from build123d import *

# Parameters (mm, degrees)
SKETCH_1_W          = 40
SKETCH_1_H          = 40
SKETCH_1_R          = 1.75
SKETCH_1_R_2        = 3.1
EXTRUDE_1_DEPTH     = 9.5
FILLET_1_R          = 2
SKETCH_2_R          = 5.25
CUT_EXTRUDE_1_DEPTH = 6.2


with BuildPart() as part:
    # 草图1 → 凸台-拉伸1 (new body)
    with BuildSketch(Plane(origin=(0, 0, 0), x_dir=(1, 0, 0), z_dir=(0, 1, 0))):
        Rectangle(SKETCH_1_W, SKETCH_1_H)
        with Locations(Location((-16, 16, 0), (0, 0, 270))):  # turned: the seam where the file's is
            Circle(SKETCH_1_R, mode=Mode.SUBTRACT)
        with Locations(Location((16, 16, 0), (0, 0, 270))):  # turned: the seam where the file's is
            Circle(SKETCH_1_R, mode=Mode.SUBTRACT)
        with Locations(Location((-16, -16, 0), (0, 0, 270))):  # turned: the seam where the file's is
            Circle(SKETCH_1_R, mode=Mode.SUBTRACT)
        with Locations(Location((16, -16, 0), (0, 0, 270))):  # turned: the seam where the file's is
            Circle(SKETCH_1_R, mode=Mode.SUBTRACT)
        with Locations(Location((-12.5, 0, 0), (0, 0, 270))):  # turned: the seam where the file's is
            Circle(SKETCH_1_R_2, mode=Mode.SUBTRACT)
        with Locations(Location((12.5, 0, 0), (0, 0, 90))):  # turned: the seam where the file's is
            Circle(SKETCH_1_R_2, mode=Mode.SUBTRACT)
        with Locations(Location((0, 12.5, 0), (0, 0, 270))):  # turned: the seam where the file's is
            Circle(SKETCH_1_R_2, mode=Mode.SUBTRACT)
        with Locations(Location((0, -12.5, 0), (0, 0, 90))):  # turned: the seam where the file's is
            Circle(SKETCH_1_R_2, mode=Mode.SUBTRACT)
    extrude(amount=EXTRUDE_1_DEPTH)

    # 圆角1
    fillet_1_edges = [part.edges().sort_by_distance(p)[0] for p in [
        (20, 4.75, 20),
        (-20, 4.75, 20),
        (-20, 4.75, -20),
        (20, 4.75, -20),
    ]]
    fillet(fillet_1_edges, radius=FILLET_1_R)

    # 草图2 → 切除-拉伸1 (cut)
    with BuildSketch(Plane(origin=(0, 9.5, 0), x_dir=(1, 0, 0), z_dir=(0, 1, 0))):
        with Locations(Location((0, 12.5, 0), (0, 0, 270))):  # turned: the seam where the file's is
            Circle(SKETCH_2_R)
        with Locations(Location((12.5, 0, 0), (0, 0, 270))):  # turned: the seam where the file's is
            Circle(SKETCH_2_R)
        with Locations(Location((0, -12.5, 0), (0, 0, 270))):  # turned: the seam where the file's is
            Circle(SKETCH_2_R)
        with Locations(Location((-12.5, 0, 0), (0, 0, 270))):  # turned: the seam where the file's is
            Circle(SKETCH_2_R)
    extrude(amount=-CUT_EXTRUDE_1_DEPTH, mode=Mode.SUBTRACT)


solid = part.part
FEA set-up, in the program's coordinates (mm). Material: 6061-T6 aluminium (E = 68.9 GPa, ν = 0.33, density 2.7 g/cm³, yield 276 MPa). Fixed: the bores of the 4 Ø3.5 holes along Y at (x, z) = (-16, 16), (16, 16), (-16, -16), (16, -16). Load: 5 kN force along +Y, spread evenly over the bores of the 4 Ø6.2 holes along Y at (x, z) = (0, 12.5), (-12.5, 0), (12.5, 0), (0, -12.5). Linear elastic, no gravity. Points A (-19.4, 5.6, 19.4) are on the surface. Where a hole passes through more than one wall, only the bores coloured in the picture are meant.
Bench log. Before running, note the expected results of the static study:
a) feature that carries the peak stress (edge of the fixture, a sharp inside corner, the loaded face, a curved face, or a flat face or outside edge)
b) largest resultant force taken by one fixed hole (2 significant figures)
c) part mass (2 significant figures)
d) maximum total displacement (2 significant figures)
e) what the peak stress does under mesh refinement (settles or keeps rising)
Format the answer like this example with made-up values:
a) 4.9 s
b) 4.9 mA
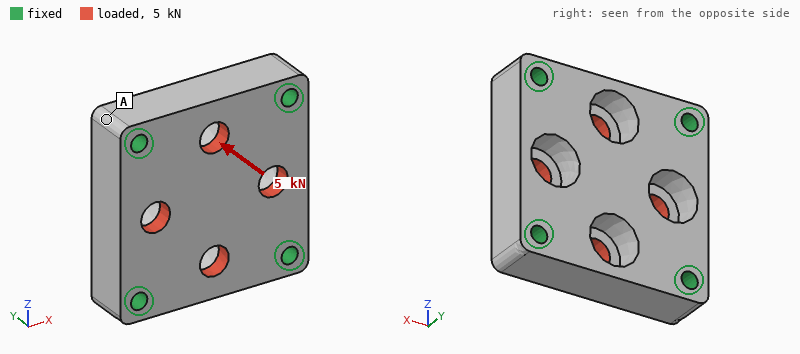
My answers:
a) edge of the fixture
b) 1.3 kN
c) 33 g
d) 16 µm
e) keeps rising
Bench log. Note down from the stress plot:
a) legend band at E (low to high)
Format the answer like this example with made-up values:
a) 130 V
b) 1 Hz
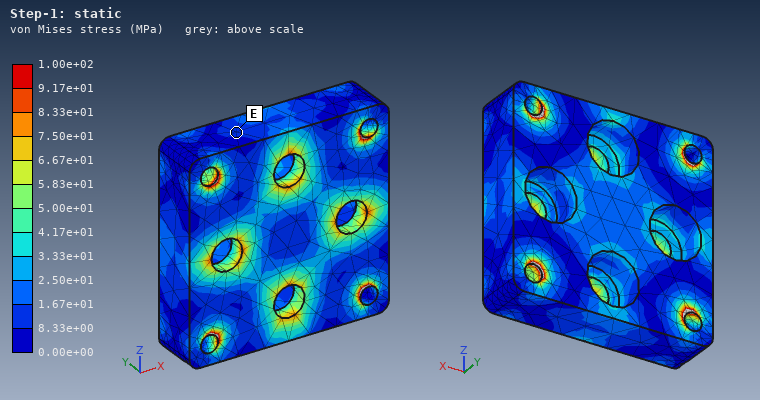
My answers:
a) 8.33e+00 to 1.67e+01 MPa
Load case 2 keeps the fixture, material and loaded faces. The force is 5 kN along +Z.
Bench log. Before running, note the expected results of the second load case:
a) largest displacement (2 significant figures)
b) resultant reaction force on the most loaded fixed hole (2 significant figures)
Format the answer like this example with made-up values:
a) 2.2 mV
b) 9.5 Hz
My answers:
a) 8.0 µm
b) 1.3 kN
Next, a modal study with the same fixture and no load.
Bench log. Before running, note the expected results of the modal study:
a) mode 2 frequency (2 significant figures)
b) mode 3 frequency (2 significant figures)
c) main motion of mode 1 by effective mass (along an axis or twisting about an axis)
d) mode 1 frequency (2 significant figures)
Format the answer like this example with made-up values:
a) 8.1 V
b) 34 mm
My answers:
a) 38 kHz
b) 38 kHz
c) along Y
d) 24 kHz
